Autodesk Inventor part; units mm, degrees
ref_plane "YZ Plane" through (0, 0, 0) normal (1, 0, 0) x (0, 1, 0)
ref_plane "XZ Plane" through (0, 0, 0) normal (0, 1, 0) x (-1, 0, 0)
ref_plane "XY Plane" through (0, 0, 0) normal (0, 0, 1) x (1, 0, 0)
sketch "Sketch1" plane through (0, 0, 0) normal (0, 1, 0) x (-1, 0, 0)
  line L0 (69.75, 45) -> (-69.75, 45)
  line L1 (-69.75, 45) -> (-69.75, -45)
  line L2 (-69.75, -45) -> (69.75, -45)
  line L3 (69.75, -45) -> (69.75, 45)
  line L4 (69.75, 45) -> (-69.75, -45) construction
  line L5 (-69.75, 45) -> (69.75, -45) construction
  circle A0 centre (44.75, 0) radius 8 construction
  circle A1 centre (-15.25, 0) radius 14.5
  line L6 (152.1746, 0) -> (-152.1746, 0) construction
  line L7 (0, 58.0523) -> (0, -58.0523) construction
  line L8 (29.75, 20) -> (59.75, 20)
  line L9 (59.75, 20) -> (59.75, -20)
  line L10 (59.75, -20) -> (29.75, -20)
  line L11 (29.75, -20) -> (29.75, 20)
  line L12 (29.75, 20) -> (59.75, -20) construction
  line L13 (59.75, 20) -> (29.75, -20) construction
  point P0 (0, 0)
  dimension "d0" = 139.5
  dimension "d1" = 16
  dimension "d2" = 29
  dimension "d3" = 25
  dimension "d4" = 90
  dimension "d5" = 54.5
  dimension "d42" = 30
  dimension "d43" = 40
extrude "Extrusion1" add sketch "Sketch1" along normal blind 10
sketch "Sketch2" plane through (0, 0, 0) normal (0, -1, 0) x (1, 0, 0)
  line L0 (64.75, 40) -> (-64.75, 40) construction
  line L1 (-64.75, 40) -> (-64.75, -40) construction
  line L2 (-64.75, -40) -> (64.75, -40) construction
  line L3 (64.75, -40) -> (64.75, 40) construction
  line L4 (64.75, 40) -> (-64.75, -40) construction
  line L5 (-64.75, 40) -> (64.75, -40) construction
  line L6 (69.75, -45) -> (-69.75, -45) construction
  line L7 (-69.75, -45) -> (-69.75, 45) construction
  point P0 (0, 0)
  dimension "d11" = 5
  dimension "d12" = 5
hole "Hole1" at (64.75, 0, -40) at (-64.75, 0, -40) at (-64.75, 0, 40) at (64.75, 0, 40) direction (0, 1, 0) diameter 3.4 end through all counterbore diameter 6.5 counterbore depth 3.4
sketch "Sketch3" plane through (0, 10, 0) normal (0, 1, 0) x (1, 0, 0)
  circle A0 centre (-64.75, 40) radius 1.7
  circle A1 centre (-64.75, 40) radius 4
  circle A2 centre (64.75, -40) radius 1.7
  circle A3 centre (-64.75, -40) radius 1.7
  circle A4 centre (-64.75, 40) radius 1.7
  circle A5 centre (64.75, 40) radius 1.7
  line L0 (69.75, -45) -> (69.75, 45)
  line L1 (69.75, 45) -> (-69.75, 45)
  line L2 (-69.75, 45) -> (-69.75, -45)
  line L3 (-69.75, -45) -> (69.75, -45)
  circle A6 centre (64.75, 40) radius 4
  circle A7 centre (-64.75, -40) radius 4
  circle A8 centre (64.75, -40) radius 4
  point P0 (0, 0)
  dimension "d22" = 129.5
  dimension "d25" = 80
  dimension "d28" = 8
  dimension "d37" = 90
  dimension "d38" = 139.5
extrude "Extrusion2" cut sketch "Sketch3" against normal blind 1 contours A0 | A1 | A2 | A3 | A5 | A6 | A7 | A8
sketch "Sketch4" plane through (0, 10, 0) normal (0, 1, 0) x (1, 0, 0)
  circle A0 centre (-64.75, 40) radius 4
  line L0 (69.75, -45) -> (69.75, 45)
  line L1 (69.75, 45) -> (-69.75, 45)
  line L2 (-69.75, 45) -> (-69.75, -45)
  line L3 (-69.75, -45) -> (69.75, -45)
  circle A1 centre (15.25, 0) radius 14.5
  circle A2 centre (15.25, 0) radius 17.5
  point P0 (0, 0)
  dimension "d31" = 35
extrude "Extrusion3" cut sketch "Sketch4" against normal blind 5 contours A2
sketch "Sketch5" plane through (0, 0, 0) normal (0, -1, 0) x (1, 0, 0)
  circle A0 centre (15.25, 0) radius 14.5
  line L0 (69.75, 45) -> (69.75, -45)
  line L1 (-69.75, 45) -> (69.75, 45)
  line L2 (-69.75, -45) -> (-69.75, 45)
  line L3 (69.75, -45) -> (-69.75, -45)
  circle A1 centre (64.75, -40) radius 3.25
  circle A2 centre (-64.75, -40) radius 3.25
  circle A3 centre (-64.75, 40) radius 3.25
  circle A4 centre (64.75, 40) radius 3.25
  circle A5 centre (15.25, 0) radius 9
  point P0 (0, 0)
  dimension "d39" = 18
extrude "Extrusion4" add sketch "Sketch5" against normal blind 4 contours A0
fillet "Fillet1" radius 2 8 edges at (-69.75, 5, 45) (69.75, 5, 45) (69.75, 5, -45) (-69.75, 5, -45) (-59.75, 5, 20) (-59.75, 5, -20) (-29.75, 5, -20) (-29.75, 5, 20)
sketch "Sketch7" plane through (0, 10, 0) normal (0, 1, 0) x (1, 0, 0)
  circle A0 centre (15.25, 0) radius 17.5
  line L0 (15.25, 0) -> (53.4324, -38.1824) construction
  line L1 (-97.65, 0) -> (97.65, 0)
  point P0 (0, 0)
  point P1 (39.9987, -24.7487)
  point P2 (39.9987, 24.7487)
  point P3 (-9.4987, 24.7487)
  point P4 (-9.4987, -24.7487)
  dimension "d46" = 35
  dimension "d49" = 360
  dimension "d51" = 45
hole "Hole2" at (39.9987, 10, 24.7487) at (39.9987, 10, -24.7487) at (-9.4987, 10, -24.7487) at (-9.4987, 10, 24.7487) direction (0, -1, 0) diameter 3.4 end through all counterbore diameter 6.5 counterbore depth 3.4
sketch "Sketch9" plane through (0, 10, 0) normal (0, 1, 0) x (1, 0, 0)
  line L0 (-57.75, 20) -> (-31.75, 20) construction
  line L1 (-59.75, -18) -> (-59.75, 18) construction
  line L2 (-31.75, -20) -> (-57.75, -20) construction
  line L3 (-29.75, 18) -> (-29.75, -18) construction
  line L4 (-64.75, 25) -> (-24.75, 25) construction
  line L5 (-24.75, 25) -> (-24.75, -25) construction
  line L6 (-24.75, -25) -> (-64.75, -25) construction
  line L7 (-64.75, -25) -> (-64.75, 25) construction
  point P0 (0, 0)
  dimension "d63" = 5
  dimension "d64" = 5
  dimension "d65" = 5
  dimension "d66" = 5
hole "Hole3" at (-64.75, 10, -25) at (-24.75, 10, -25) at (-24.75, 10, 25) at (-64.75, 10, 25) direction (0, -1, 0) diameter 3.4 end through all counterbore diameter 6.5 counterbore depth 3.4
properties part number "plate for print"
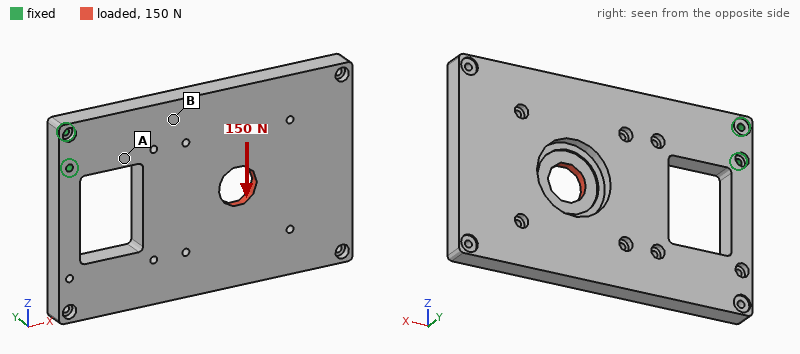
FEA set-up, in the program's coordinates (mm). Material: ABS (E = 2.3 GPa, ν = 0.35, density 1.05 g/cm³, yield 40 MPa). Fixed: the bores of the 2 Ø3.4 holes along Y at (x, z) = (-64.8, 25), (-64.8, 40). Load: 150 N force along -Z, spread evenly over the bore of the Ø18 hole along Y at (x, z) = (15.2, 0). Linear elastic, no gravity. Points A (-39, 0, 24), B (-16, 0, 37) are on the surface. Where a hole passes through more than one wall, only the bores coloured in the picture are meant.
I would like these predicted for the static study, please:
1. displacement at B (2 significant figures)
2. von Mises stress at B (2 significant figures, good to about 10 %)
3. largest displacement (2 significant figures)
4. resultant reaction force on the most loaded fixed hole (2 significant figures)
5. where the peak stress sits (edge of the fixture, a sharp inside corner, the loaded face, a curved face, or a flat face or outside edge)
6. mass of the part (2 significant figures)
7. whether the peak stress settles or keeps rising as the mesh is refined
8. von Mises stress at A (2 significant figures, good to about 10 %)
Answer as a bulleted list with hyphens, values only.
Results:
- 0.52 mm
- 1.4 MPa
- 1.9 mm
- 690 N
- edge of the fixture
- 110 g
- keeps rising
- 3.4 MPa
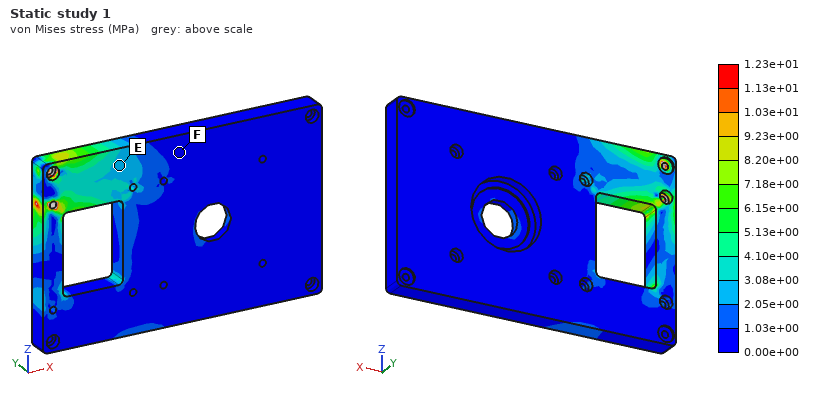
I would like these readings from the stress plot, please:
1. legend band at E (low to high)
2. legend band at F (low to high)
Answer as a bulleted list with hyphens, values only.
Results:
- 2.05e+00 to 3.08e+00 MPa
- 0.00e+00 to 1.03e+00 MPa
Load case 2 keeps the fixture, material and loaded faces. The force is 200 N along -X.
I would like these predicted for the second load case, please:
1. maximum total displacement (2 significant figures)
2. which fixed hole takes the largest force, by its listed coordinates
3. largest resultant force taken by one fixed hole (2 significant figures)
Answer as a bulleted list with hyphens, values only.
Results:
- 1.1 mm
- (-64.8, 25)
- 470 N
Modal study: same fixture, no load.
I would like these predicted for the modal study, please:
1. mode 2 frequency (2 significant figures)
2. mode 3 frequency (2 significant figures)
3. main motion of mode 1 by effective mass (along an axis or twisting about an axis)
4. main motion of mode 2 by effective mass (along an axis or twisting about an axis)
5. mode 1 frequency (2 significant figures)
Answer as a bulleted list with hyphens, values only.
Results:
- 180 Hz
- 200 Hz
- along Y
- along Z
- 67 Hz
